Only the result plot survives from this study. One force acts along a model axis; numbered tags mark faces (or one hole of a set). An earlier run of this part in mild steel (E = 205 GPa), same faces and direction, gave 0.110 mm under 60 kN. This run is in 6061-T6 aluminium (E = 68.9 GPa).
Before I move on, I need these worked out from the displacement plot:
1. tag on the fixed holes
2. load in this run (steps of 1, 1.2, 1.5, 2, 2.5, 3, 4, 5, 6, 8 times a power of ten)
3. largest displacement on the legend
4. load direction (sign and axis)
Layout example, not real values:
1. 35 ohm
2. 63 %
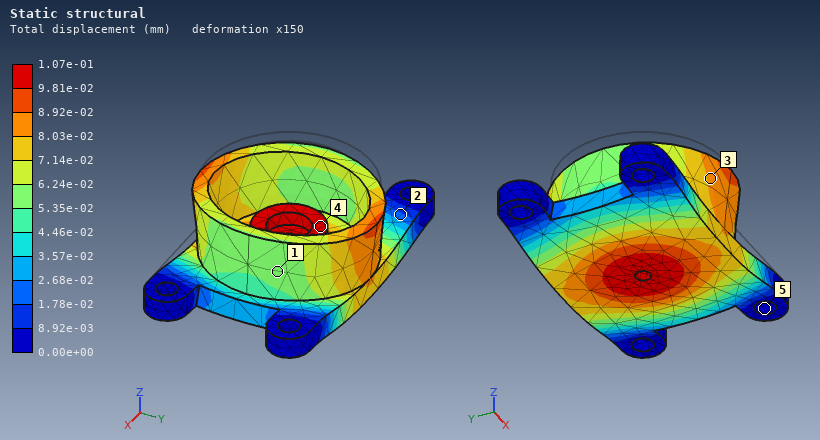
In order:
1. 5
2. 20 kN
3. 1.07e-01 mm
4. -Z
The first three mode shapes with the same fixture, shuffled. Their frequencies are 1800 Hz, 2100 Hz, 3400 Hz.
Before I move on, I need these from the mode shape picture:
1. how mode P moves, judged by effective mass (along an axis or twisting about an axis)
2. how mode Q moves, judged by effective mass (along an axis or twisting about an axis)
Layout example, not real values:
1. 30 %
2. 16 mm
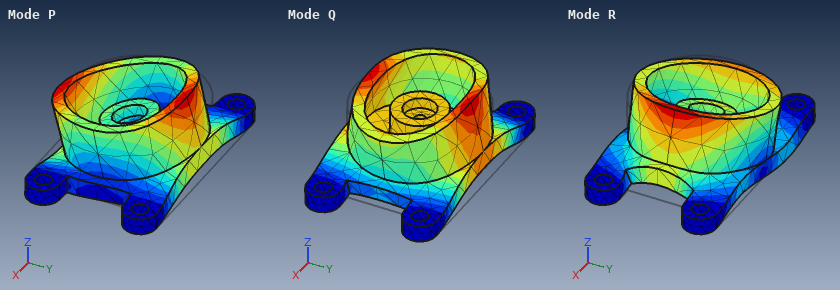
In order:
1. along Y
2. along Z
